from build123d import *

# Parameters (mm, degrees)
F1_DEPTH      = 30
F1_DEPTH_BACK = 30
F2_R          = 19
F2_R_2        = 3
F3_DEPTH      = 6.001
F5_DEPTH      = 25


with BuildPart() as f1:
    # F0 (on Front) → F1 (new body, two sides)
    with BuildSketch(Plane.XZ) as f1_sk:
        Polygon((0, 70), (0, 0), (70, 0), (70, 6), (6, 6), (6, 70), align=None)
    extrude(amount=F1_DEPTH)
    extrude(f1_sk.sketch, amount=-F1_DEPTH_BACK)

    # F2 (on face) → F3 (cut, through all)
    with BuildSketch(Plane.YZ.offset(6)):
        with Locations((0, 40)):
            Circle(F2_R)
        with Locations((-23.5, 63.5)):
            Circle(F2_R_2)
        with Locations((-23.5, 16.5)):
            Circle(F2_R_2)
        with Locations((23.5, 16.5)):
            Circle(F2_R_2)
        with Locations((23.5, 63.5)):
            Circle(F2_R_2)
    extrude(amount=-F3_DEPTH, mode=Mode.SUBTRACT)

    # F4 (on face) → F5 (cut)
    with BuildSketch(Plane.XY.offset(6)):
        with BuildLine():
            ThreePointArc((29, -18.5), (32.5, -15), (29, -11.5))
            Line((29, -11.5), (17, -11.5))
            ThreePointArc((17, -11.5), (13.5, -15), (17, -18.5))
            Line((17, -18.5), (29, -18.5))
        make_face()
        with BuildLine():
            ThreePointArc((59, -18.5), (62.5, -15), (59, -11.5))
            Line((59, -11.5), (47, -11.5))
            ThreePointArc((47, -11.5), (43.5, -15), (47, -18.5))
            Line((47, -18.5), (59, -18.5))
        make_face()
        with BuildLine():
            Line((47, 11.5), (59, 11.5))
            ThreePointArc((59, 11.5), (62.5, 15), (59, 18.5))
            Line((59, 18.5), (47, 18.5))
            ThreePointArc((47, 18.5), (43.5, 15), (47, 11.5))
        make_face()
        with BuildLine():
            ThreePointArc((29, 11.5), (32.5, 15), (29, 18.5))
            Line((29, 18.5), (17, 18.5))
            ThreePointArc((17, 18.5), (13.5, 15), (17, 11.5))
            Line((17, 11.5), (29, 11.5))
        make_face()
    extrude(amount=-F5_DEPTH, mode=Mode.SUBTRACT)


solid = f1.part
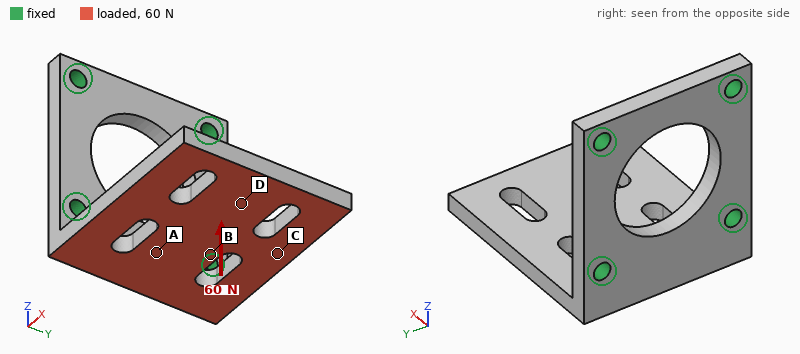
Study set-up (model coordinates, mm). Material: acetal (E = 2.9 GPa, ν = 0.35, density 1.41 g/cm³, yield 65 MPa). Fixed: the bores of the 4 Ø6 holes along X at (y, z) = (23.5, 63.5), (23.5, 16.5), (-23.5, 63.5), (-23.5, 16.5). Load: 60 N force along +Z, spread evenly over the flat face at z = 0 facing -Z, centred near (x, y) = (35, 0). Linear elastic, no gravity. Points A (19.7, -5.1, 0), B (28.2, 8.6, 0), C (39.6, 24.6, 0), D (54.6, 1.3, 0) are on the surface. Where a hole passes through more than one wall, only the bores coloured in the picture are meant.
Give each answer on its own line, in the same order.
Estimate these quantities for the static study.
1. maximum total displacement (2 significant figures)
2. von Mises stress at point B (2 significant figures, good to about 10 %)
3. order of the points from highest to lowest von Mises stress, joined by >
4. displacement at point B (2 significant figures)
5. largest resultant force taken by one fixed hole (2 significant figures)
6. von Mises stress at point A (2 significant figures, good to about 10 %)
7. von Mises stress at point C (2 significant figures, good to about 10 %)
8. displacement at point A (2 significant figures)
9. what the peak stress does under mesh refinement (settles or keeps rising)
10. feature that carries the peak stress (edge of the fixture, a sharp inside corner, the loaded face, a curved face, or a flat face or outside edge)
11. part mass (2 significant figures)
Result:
1.3 mm
2.5 MPa
A > B > C > D
0.37 mm
32 N
3.5 MPa
1.3 MPa
0.23 mm
keeps rising
edge of the fixture
53 g
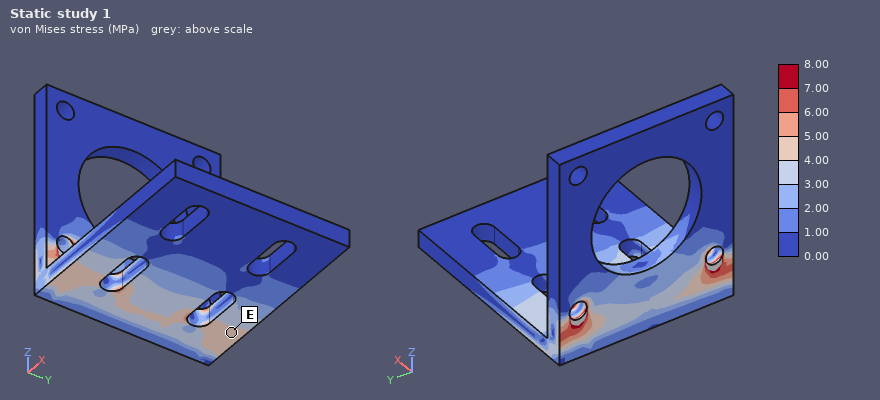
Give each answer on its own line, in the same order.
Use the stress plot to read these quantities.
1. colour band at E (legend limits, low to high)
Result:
4.00 to 5.00 MPa
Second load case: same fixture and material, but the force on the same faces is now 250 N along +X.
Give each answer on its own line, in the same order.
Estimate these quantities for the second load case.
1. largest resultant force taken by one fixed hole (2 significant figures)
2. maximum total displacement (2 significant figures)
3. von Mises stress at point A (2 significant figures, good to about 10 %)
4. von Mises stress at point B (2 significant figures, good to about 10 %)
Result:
130 N
1.1 mm
2.2 MPa
1.8 MPa
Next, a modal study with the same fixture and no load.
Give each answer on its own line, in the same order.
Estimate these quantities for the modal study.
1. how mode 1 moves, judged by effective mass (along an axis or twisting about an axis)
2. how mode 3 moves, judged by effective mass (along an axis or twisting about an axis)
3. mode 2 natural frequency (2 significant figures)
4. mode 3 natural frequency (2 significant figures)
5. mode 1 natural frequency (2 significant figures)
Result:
along Z
along Y
670 Hz
990 Hz
240 Hz
